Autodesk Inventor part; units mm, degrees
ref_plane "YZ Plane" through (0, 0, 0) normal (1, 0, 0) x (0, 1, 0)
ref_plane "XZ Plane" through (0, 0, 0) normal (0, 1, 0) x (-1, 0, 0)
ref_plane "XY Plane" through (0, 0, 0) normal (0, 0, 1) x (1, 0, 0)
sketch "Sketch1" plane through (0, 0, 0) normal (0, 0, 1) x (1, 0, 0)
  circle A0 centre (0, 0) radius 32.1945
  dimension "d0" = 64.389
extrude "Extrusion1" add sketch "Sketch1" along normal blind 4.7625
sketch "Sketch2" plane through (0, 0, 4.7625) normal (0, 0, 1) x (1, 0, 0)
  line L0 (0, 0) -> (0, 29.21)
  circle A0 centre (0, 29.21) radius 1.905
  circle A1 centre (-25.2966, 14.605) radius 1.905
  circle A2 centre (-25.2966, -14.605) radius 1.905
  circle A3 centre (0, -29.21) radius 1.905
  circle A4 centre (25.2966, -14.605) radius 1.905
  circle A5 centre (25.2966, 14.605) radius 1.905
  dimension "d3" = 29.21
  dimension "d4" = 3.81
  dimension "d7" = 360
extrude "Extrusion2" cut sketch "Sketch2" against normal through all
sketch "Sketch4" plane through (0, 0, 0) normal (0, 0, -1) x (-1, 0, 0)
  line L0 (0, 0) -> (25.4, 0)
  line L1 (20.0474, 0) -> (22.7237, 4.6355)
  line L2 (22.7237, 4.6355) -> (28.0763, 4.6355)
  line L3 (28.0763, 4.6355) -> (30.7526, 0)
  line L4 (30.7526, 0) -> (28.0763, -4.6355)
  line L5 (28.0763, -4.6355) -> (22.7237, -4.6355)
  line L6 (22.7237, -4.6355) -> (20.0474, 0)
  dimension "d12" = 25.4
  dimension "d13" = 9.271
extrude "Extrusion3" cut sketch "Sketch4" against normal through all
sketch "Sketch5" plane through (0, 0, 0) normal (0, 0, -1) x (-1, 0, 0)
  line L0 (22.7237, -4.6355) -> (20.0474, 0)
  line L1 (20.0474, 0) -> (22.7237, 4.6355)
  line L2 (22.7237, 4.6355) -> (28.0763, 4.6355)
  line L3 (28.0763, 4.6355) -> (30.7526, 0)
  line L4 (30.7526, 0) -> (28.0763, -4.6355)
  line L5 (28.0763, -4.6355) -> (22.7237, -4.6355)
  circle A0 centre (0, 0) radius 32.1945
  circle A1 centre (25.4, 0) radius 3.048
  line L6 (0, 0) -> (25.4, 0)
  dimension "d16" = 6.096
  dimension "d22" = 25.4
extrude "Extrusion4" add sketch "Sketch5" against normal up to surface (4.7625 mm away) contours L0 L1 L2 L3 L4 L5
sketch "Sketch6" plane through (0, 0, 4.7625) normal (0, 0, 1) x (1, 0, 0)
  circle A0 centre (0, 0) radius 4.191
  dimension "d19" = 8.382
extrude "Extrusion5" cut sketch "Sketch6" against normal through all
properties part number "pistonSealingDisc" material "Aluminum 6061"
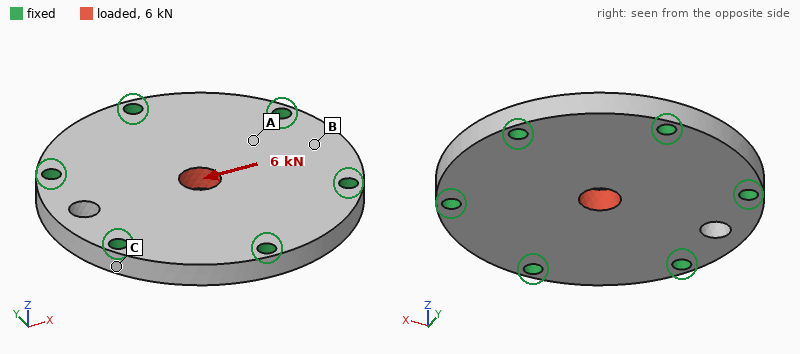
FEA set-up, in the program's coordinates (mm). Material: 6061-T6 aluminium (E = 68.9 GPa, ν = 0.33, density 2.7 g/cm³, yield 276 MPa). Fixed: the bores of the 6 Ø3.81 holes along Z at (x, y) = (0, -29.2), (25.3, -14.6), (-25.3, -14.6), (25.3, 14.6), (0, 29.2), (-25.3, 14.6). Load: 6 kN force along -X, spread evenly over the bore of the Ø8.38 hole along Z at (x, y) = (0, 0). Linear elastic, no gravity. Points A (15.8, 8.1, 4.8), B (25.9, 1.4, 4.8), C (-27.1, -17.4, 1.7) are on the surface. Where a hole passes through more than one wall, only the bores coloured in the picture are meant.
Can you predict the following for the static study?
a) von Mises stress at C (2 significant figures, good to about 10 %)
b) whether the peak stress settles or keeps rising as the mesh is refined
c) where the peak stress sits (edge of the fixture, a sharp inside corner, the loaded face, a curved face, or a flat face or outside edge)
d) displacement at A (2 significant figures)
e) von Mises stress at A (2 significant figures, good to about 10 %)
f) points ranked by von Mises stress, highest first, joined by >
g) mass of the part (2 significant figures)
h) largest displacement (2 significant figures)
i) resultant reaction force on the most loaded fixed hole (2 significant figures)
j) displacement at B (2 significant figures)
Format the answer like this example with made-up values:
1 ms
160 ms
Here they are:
15 MPa
keeps rising
a sharp inside corner
4.5 µm
24 MPa
A > C > B
40 g
12 µm
1.4 kN
4.6 µm
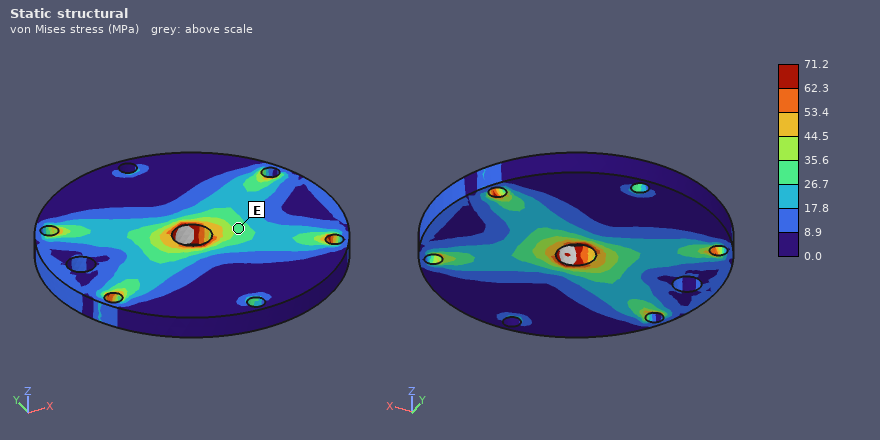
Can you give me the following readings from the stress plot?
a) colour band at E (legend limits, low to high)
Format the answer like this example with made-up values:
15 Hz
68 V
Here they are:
26.7 to 35.6 MPa
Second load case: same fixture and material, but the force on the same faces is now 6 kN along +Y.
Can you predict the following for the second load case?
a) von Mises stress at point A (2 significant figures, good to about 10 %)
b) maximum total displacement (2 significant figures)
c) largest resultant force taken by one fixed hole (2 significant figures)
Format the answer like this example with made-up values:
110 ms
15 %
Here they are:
15 MPa
12 µm
1.5 kN
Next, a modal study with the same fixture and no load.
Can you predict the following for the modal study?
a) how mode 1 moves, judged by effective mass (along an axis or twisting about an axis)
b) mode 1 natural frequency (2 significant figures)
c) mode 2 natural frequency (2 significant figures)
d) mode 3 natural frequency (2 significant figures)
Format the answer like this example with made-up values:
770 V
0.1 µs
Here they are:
along Z
11 kHz
21 kHz
21 kHz
